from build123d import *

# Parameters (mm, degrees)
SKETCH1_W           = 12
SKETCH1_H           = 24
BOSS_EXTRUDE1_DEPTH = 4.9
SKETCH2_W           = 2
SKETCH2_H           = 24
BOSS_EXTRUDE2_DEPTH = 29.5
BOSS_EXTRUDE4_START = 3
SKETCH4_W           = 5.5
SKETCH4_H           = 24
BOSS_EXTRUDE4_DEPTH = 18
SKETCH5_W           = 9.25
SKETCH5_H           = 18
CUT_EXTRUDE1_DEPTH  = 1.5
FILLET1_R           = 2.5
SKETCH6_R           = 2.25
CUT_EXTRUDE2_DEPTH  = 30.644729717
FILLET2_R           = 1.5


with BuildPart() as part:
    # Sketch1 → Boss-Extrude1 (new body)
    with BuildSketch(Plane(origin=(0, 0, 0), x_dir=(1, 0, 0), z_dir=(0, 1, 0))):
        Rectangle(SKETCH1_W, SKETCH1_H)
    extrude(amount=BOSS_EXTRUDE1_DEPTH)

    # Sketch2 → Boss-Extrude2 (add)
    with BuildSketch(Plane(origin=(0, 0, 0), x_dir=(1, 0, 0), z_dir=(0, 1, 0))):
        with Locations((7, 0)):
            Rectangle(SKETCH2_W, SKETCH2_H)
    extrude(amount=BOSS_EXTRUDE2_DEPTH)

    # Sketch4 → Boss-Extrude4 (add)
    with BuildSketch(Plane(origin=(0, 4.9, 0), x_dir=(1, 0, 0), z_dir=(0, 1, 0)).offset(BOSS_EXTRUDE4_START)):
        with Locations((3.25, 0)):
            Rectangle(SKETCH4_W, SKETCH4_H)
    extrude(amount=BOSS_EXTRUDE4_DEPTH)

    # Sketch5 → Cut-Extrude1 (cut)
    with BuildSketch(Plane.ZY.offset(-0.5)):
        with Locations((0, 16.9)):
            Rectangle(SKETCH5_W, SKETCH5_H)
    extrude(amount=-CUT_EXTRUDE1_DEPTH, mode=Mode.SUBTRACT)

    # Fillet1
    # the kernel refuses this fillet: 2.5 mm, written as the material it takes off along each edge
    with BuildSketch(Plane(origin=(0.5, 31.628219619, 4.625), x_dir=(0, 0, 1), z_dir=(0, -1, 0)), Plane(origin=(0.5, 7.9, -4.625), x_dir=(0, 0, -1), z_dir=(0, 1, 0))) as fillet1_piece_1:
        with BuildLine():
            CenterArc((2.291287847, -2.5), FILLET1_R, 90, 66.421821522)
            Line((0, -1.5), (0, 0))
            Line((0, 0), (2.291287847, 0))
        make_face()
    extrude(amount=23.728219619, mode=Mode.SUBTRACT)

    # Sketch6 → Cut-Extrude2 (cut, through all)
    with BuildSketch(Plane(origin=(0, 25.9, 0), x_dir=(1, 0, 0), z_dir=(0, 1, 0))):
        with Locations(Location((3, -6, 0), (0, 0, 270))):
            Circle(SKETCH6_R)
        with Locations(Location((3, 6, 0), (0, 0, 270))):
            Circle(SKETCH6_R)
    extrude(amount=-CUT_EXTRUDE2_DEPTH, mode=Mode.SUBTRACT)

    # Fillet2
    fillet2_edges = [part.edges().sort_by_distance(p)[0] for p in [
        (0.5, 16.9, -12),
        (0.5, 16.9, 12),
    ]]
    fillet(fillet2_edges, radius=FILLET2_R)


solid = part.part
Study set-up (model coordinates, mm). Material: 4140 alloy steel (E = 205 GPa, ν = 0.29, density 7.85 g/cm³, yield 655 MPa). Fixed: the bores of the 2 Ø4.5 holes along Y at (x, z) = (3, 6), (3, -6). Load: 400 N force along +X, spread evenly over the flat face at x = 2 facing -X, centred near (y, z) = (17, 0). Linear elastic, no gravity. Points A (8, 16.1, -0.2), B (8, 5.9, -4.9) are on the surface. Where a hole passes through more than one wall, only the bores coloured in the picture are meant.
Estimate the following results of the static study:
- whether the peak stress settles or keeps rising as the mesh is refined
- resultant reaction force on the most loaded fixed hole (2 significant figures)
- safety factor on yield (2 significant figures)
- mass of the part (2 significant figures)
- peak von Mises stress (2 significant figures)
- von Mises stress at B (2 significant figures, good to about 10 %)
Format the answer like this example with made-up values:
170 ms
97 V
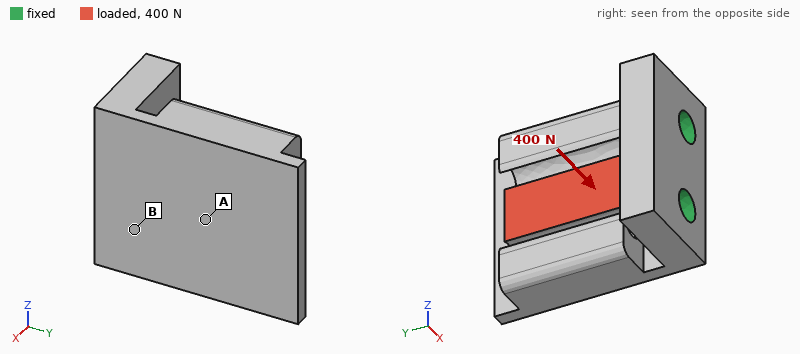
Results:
settles
200 N
2.5
33 g
260 MPa
240 MPa
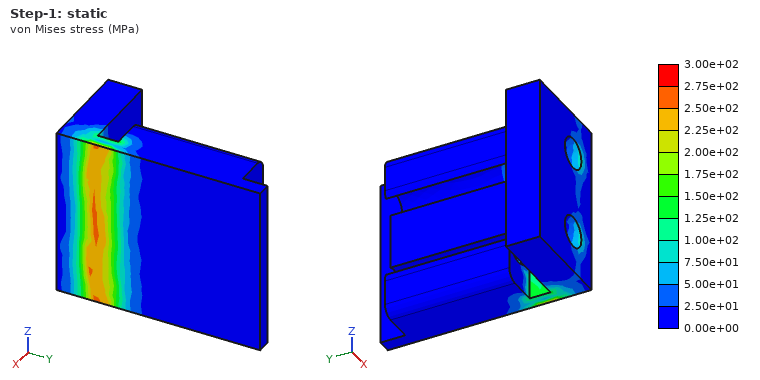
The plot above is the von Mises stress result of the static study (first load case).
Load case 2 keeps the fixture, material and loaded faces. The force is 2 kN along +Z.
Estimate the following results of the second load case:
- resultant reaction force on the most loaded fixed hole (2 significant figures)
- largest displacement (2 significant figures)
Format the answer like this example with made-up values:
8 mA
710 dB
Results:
2.0 kN
44 µm
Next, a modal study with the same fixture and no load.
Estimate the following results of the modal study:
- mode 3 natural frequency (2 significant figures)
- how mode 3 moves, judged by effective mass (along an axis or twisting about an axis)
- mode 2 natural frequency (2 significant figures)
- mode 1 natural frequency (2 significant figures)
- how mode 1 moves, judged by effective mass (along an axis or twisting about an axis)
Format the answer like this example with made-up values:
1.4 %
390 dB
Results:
12 kHz
along Z
8600 Hz
2200 Hz
along X
